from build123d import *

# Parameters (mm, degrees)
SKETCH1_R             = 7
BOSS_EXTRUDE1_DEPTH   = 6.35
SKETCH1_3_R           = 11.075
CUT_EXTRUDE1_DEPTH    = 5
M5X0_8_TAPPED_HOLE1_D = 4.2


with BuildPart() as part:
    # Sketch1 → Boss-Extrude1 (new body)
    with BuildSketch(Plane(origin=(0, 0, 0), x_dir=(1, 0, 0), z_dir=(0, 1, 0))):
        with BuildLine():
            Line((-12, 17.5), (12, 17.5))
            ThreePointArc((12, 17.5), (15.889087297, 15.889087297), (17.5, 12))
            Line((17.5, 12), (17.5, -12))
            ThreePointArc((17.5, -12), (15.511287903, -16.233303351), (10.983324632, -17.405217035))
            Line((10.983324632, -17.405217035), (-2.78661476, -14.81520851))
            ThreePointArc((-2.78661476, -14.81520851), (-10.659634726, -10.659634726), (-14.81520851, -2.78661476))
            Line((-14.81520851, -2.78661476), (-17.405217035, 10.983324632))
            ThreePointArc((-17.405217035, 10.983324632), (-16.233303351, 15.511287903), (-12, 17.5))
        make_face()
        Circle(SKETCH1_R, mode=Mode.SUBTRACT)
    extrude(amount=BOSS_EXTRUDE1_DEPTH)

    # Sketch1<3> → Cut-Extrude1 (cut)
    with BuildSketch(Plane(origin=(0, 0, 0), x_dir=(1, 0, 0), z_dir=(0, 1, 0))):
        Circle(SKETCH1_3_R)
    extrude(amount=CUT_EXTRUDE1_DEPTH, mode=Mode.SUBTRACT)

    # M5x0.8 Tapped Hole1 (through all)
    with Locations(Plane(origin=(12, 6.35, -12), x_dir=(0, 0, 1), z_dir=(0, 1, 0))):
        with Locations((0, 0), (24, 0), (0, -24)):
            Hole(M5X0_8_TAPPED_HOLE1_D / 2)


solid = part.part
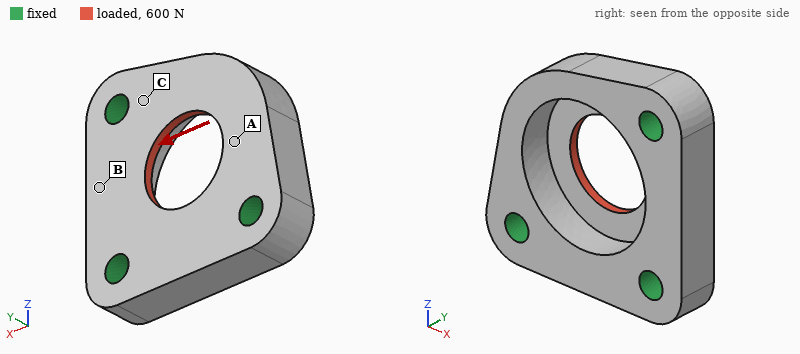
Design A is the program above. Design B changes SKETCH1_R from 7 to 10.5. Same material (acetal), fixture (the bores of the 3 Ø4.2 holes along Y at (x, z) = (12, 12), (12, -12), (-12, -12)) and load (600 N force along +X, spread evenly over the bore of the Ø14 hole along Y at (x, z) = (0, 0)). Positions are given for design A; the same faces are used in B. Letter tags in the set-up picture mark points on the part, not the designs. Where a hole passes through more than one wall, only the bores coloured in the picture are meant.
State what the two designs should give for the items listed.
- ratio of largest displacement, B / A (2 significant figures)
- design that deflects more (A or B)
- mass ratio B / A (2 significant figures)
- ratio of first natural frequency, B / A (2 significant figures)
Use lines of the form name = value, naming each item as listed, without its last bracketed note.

ratio of largest displacement, B / A = 1.4
design that deflects more = B
mass ratio B / A = 0.94
ratio of first natural frequency, B / A = 0.99
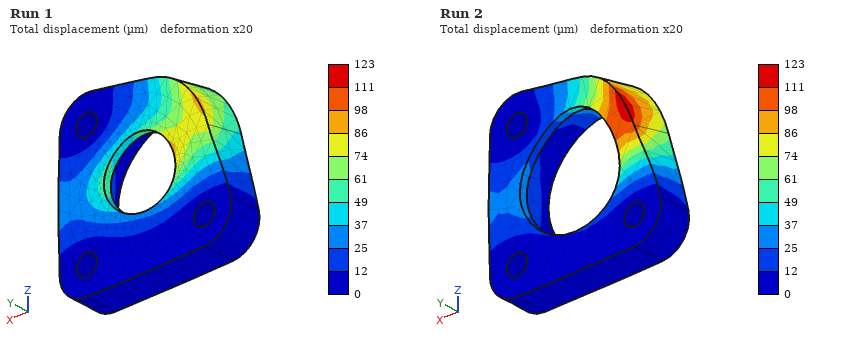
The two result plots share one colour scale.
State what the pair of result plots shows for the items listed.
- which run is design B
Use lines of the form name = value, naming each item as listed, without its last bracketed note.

which run is design B = Run 2
